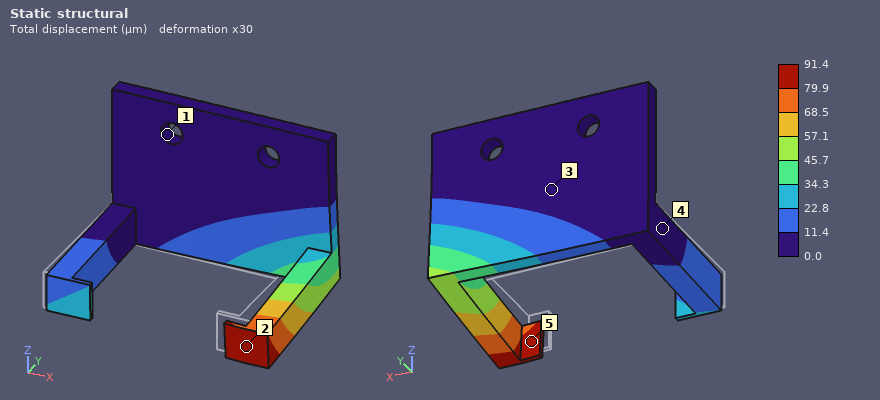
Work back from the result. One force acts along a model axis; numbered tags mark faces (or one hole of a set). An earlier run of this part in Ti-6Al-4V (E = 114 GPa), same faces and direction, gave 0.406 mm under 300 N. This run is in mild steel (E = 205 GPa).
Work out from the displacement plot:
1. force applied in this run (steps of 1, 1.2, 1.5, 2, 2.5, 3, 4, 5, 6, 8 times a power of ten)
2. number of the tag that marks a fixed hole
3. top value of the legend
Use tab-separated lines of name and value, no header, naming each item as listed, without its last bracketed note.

force applied in this run	120 N
number of the tag that marks a fixed hole	1
top value of the legend	91.4 µm
